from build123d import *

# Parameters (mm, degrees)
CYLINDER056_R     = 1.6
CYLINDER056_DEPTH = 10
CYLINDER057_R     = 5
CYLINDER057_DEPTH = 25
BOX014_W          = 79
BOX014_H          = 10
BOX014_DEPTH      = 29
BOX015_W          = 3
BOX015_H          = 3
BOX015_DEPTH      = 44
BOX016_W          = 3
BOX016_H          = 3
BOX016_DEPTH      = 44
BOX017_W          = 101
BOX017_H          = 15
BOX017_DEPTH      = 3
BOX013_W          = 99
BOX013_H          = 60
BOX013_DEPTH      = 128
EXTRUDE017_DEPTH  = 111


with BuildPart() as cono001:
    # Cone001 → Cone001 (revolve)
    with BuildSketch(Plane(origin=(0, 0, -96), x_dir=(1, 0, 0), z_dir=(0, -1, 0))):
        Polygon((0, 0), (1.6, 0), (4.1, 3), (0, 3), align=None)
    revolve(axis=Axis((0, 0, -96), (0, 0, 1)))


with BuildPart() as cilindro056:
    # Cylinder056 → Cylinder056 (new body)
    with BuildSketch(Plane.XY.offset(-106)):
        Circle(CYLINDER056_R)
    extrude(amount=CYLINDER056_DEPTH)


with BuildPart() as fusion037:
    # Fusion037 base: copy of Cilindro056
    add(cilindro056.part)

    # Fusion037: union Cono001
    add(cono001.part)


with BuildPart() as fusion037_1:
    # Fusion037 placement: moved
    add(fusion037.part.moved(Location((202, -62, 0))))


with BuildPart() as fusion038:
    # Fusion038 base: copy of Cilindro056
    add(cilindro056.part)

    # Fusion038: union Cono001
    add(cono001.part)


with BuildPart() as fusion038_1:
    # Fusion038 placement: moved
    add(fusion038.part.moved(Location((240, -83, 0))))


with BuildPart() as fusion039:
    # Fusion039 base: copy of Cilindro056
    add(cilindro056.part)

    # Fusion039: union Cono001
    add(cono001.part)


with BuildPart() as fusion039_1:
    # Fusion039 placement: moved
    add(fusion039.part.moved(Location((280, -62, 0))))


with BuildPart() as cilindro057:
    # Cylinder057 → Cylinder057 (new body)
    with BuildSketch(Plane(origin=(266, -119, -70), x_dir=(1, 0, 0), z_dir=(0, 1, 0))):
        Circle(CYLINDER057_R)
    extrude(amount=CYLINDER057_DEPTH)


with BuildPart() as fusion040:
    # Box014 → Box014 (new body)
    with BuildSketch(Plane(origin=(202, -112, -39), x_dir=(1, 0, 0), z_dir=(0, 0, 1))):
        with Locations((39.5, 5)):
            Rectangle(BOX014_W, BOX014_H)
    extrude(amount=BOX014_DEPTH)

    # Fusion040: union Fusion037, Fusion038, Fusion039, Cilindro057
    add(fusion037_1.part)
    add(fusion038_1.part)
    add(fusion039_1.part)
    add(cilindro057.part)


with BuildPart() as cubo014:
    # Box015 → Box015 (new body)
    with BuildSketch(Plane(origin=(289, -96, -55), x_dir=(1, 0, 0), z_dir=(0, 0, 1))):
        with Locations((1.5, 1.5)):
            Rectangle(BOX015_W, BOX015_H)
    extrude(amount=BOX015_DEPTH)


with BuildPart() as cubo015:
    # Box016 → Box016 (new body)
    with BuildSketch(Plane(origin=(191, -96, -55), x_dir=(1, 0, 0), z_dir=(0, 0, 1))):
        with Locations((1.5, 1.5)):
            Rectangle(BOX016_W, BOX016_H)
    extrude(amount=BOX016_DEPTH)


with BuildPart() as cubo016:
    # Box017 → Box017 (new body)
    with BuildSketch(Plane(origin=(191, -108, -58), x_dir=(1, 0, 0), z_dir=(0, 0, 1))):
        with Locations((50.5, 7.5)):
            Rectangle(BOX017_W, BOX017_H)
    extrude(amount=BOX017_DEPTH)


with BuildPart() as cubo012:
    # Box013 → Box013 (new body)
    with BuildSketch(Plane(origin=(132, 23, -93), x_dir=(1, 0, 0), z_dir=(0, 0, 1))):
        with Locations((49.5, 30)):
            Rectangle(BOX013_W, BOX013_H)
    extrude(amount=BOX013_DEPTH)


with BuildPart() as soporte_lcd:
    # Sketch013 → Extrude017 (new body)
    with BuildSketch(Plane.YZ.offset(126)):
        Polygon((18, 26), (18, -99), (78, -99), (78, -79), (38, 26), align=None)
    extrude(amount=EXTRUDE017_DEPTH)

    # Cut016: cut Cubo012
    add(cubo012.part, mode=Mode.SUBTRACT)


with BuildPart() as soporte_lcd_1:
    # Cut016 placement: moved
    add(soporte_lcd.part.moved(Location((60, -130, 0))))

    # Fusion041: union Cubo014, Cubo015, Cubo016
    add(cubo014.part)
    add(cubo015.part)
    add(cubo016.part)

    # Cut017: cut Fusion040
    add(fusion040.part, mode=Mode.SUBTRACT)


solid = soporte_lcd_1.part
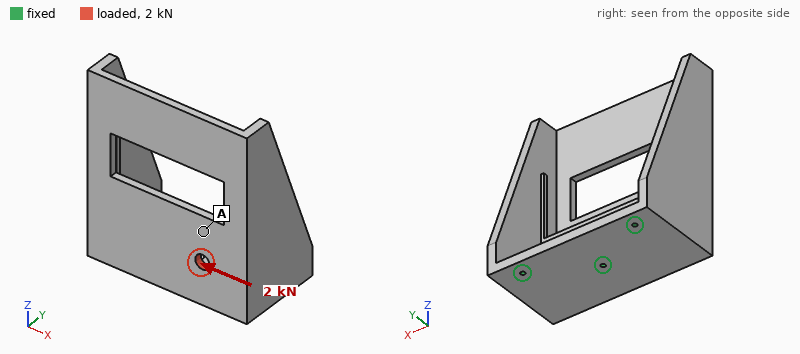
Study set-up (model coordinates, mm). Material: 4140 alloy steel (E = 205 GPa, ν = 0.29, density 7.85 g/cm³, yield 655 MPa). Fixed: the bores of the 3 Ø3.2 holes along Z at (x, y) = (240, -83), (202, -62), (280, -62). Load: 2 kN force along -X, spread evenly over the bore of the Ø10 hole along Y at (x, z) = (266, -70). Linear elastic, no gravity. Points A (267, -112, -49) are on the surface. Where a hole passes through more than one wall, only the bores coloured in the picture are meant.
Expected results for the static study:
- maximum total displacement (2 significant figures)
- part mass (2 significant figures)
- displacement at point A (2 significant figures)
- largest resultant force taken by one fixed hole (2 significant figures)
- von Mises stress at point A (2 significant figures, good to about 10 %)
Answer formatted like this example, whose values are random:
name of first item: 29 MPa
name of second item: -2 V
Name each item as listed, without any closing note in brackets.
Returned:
maximum total displacement: 0.17 mm
part mass: 1.2 kg
displacement at point A: 0.055 mm
largest resultant force taken by one fixed hole: 1.2 kN
von Mises stress at point A: 9.9 MPa
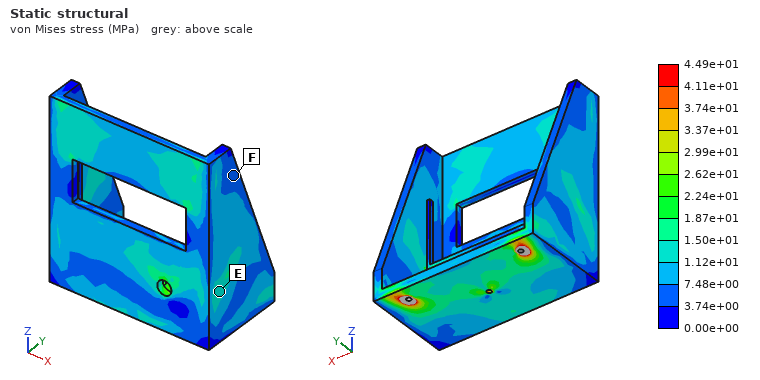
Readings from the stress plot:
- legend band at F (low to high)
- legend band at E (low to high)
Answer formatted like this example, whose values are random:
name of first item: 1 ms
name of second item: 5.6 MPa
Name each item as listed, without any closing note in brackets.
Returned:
legend band at F: 3.74e+00 to 7.48e+00 MPa
legend band at E: 1.12e+01 to 1.50e+01 MPa
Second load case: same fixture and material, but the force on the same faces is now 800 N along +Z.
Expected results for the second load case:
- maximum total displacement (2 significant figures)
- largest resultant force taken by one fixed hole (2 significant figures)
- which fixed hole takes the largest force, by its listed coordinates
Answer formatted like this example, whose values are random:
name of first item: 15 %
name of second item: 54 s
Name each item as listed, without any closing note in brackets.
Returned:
maximum total displacement: 0.16 mm
largest resultant force taken by one fixed hole: 1.3 kN
which fixed hole takes the largest force, by its listed coordinates: (240, -83)
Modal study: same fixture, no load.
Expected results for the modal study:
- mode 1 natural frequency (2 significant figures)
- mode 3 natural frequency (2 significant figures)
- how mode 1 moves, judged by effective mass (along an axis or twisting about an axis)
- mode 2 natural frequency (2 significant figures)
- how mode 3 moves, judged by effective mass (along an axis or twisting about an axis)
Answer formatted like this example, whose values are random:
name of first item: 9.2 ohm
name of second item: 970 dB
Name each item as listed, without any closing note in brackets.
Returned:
mode 1 natural frequency: 430 Hz
mode 3 natural frequency: 1600 Hz
how mode 1 moves, judged by effective mass: along X
mode 2 natural frequency: 450 Hz
how mode 3 moves, judged by effective mass: along Z
